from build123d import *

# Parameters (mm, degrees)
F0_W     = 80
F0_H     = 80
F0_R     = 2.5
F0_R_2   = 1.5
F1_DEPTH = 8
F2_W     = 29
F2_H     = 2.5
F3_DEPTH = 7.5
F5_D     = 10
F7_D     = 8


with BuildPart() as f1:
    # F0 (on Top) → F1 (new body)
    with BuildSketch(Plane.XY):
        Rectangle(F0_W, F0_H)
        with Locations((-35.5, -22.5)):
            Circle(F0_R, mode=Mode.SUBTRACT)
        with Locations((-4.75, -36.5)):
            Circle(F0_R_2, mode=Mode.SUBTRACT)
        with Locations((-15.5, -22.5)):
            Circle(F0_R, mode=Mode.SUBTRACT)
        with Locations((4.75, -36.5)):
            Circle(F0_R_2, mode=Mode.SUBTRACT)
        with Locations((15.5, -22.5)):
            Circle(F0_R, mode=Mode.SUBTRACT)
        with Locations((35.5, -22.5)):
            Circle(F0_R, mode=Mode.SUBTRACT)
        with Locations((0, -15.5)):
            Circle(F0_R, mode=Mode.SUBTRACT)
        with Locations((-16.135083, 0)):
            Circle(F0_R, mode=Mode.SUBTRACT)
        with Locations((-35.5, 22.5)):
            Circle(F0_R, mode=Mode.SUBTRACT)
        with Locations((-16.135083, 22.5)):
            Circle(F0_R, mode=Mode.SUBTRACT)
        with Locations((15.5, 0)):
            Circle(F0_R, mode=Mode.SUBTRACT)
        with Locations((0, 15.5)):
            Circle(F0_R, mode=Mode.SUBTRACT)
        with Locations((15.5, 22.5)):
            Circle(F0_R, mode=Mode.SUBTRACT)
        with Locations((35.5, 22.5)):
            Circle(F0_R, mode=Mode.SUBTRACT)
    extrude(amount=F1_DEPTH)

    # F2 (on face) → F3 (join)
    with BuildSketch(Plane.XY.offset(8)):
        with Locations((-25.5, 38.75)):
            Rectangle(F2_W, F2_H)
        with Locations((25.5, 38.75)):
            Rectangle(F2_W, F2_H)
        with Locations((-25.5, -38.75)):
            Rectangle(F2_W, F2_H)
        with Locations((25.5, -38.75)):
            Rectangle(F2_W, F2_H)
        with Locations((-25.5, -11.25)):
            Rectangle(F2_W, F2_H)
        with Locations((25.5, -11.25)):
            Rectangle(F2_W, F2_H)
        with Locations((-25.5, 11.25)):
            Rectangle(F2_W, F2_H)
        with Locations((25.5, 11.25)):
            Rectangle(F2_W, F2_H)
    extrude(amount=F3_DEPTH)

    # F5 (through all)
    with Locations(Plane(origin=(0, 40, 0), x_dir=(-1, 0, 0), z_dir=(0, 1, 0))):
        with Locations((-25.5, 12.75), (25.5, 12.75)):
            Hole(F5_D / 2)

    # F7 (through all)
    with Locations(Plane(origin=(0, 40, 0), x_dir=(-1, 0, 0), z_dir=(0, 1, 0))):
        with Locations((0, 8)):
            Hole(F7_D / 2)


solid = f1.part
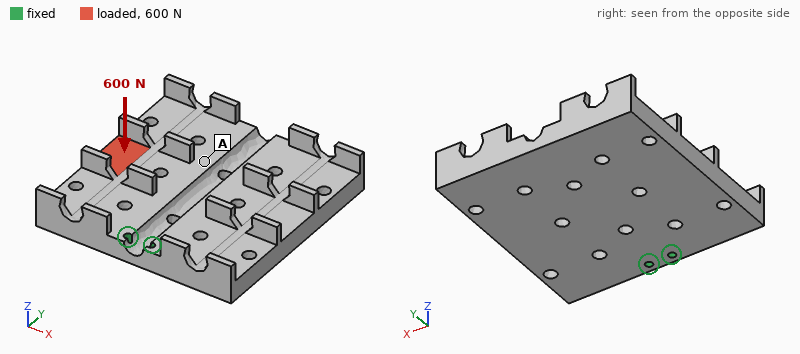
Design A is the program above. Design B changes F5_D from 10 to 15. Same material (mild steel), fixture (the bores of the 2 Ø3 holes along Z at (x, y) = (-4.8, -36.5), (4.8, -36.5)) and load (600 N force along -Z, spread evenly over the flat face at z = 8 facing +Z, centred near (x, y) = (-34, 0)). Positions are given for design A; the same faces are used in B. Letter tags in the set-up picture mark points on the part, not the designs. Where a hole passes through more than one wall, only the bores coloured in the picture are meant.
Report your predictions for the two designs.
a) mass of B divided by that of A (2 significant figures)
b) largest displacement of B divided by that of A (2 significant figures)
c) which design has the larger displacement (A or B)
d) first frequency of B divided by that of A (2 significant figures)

0.91
1.1
B
1.0
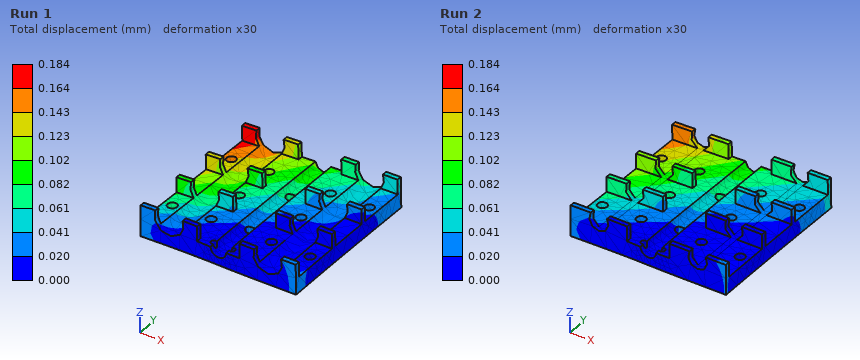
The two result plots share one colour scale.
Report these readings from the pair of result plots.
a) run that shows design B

Run 1
